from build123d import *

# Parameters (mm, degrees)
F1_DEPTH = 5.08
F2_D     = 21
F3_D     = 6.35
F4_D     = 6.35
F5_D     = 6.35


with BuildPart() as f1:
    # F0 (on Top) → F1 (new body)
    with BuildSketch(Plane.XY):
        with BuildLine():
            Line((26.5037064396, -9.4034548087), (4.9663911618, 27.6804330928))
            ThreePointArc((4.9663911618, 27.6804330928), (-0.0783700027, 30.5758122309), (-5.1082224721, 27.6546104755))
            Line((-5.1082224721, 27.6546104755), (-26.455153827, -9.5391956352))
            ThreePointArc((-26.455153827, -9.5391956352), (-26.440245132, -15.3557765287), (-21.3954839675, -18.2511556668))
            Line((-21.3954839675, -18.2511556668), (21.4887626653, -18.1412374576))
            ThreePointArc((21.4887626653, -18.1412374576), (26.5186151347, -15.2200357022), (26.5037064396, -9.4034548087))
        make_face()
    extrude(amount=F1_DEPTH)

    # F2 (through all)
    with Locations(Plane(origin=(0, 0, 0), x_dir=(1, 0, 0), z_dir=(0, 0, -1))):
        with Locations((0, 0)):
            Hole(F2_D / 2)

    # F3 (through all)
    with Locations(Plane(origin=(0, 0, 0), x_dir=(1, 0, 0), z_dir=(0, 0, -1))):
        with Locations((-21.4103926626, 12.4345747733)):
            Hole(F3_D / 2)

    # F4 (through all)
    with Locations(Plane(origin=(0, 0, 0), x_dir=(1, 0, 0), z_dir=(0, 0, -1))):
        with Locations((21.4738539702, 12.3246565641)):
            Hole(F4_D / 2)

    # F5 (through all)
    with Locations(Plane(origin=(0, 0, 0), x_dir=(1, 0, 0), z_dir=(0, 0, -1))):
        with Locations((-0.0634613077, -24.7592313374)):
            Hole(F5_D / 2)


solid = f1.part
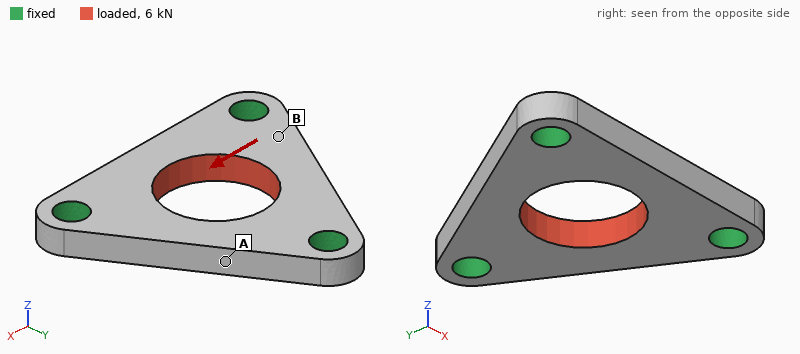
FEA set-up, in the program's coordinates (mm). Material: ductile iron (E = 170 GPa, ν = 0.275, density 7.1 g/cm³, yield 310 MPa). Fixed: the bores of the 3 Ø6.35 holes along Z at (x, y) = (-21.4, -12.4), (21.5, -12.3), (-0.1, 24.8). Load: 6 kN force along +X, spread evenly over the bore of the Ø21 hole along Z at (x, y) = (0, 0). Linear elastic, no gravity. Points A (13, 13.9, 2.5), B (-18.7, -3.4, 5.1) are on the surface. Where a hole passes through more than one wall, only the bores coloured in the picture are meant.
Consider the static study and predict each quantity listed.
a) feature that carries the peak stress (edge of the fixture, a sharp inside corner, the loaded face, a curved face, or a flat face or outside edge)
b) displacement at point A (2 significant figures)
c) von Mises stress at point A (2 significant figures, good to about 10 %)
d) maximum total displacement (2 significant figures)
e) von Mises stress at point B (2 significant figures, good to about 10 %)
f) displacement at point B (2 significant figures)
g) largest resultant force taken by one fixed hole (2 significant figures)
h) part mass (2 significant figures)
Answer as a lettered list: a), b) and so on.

a) edge of the fixture
b) 7.9 µm
c) 52 MPa
d) 9.4 µm
e) 25 MPa
f) 3.3 µm
g) 2.1 kN
h) 44 g
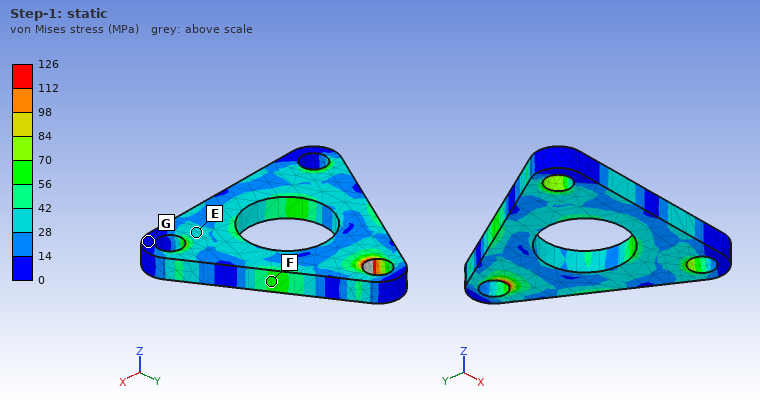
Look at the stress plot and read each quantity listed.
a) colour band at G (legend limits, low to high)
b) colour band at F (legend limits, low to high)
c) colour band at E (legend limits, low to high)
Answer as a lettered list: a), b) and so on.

a) 0 to 14 MPa
b) 56 to 70 MPa
c) 28 to 42 MPa
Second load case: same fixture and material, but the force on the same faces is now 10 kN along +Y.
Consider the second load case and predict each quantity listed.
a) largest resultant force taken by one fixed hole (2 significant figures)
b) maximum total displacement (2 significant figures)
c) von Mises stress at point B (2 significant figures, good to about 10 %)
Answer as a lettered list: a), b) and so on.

a) 3.5 kN
b) 18 µm
c) 54 MPa
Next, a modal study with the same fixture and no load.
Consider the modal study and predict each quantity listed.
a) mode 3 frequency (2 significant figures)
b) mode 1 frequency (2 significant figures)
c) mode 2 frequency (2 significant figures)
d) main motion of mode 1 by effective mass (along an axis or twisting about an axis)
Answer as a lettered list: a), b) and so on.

a) 18 kHz
b) 16 kHz
c) 18 kHz
d) along Z
